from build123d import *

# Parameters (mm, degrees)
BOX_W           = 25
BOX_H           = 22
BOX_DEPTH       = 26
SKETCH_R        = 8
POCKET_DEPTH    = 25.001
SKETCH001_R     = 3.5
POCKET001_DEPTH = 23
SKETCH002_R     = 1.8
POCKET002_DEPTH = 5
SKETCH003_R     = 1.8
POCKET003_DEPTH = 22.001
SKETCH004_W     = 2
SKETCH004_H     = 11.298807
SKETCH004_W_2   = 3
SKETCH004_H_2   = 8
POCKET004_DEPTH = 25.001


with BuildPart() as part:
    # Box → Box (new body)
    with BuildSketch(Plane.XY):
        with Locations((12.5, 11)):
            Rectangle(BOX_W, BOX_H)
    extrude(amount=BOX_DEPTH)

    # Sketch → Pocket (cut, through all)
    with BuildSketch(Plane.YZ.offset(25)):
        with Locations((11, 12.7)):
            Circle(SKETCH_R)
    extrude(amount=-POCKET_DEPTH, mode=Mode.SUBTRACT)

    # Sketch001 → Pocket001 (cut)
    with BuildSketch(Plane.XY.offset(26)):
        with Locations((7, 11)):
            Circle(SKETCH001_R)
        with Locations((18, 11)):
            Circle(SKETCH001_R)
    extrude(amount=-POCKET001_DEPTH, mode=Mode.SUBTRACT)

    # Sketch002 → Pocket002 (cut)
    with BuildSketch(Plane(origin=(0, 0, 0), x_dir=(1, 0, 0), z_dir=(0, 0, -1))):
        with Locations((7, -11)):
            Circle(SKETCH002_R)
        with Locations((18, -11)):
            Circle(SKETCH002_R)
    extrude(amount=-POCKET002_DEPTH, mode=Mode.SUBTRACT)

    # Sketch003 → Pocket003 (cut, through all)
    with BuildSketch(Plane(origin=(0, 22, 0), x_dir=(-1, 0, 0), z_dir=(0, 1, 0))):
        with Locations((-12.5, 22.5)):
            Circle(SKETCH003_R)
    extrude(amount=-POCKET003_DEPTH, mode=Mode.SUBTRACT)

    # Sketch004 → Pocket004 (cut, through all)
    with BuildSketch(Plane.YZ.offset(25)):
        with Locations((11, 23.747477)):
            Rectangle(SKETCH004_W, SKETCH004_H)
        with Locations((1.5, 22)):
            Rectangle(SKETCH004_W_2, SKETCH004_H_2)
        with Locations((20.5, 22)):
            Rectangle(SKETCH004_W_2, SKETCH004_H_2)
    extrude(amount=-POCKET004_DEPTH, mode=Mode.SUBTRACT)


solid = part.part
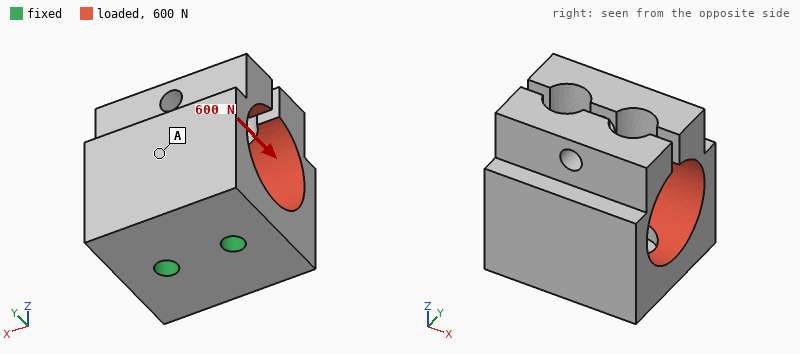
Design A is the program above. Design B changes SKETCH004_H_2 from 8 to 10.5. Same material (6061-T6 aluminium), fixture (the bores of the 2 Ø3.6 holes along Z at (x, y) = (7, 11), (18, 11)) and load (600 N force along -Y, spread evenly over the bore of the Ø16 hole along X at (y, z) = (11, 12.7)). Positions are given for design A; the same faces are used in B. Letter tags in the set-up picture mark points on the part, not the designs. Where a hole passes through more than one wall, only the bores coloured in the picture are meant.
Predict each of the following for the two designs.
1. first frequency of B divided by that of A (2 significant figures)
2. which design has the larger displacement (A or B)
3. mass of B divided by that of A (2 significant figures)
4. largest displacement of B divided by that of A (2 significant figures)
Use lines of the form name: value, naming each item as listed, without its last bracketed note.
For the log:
first frequency of B divided by that of A: 0.89
which design has the larger displacement: B
mass of B divided by that of A: 0.97
largest displacement of B divided by that of A: 1.2
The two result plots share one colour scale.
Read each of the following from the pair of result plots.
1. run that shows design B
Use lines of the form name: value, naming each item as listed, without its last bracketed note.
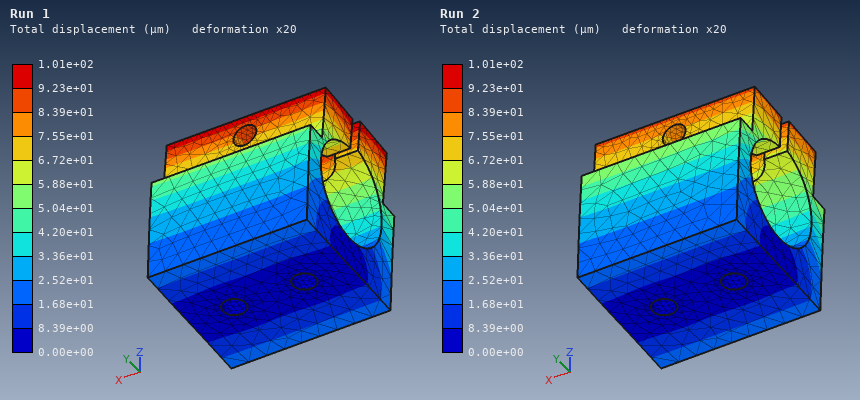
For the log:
run that shows design B: Run 1
